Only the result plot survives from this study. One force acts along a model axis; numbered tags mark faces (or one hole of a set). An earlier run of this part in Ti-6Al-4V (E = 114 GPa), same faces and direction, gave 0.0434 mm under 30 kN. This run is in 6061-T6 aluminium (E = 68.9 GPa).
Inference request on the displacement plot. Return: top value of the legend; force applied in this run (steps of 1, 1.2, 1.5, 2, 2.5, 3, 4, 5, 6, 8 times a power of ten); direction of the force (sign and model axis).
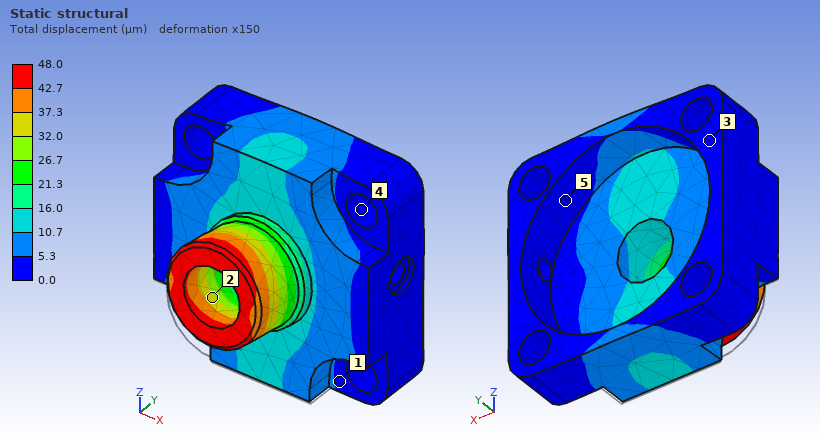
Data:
48.0 µm
20 kN
+Z
